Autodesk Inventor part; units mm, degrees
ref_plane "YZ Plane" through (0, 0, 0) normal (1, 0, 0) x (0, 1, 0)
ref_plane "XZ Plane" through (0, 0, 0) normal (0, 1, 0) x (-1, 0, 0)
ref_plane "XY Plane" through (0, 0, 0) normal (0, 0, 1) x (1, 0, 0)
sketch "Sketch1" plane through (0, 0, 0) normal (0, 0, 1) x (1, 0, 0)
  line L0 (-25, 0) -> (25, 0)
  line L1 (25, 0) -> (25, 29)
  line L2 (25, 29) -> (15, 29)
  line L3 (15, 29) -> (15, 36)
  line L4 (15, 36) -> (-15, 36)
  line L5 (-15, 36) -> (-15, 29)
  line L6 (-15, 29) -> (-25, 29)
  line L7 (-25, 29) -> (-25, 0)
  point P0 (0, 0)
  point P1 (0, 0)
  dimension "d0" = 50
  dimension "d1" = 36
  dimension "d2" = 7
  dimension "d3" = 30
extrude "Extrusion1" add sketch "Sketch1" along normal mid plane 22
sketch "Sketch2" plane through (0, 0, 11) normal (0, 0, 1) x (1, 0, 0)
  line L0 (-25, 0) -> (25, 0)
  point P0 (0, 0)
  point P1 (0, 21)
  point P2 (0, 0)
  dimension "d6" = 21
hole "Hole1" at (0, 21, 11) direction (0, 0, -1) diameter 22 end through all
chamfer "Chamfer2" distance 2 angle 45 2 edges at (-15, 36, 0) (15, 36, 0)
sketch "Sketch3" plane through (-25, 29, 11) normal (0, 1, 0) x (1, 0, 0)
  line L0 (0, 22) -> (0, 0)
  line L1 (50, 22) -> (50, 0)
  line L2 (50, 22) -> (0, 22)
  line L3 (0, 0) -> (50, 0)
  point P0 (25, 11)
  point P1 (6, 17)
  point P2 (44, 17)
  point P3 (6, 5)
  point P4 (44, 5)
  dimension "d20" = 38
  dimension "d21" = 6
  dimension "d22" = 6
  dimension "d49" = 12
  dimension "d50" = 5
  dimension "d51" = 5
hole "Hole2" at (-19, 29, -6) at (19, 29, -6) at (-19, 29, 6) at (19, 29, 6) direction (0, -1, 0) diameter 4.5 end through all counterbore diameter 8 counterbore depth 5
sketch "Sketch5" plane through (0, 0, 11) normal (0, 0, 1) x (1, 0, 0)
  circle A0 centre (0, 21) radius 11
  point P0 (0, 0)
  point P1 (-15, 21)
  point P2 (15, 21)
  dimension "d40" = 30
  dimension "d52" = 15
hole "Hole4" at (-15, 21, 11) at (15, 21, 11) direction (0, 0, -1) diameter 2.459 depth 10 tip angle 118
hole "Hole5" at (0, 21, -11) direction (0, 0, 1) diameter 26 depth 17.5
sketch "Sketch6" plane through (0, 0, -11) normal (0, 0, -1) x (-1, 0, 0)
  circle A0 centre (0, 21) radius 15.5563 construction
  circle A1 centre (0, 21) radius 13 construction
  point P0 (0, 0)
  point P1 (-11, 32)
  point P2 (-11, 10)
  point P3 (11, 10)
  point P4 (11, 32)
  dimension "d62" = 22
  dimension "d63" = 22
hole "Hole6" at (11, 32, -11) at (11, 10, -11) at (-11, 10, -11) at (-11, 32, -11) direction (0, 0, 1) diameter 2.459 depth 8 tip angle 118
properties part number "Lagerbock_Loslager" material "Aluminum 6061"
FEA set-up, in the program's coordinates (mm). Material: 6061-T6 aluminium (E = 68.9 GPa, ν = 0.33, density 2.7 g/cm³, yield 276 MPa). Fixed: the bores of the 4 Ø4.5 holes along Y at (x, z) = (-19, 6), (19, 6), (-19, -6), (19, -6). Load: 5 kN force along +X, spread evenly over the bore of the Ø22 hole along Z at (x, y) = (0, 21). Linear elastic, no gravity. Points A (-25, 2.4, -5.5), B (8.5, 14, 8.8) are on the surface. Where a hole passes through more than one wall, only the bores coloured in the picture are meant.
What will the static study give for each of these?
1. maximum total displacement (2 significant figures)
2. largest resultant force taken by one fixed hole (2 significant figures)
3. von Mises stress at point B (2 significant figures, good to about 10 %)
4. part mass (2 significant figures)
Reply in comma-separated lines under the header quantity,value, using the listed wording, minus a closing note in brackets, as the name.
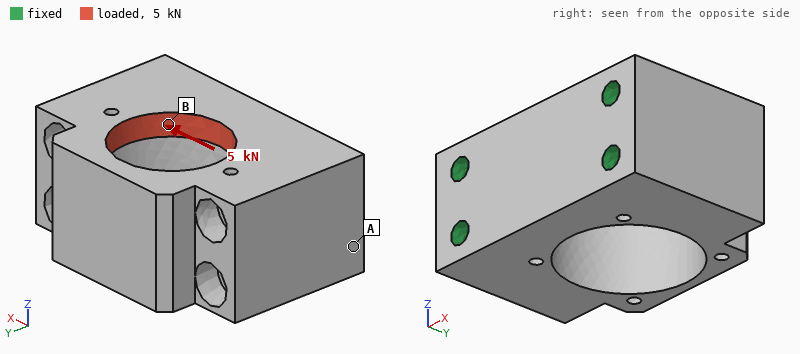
quantity,value
maximum total displacement,16 µm
largest resultant force taken by one fixed hole,2.1 kN
von Mises stress at point B,22 MPa
part mass,61 g
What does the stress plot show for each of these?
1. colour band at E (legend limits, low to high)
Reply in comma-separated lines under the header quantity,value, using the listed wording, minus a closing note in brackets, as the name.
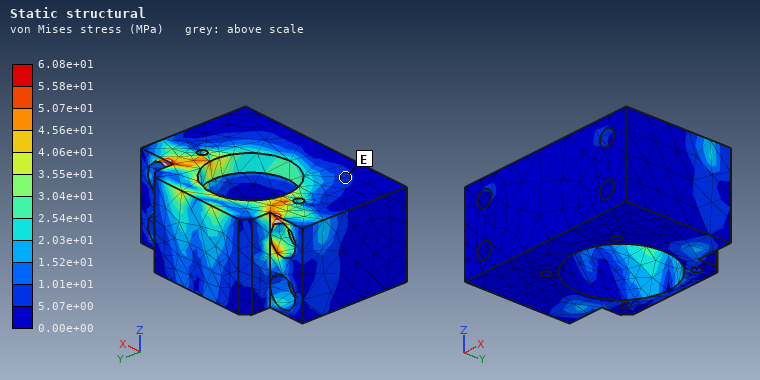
quantity,value
colour band at E,5.07e+00 to 1.01e+01 MPa
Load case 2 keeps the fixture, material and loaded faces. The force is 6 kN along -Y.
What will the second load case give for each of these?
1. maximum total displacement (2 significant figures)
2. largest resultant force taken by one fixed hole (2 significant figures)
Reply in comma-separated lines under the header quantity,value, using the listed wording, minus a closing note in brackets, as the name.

quantity,value
maximum total displacement,28 µm
largest resultant force taken by one fixed hole,2.9 kN
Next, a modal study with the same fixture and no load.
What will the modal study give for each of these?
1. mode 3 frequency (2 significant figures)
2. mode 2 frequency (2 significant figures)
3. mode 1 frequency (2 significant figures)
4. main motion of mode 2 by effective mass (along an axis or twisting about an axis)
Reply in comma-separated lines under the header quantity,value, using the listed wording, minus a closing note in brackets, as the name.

quantity,value
mode 3 frequency,30 kHz
mode 2 frequency,23 kHz
mode 1 frequency,22 kHz
main motion of mode 2 by effective mass,along Z
